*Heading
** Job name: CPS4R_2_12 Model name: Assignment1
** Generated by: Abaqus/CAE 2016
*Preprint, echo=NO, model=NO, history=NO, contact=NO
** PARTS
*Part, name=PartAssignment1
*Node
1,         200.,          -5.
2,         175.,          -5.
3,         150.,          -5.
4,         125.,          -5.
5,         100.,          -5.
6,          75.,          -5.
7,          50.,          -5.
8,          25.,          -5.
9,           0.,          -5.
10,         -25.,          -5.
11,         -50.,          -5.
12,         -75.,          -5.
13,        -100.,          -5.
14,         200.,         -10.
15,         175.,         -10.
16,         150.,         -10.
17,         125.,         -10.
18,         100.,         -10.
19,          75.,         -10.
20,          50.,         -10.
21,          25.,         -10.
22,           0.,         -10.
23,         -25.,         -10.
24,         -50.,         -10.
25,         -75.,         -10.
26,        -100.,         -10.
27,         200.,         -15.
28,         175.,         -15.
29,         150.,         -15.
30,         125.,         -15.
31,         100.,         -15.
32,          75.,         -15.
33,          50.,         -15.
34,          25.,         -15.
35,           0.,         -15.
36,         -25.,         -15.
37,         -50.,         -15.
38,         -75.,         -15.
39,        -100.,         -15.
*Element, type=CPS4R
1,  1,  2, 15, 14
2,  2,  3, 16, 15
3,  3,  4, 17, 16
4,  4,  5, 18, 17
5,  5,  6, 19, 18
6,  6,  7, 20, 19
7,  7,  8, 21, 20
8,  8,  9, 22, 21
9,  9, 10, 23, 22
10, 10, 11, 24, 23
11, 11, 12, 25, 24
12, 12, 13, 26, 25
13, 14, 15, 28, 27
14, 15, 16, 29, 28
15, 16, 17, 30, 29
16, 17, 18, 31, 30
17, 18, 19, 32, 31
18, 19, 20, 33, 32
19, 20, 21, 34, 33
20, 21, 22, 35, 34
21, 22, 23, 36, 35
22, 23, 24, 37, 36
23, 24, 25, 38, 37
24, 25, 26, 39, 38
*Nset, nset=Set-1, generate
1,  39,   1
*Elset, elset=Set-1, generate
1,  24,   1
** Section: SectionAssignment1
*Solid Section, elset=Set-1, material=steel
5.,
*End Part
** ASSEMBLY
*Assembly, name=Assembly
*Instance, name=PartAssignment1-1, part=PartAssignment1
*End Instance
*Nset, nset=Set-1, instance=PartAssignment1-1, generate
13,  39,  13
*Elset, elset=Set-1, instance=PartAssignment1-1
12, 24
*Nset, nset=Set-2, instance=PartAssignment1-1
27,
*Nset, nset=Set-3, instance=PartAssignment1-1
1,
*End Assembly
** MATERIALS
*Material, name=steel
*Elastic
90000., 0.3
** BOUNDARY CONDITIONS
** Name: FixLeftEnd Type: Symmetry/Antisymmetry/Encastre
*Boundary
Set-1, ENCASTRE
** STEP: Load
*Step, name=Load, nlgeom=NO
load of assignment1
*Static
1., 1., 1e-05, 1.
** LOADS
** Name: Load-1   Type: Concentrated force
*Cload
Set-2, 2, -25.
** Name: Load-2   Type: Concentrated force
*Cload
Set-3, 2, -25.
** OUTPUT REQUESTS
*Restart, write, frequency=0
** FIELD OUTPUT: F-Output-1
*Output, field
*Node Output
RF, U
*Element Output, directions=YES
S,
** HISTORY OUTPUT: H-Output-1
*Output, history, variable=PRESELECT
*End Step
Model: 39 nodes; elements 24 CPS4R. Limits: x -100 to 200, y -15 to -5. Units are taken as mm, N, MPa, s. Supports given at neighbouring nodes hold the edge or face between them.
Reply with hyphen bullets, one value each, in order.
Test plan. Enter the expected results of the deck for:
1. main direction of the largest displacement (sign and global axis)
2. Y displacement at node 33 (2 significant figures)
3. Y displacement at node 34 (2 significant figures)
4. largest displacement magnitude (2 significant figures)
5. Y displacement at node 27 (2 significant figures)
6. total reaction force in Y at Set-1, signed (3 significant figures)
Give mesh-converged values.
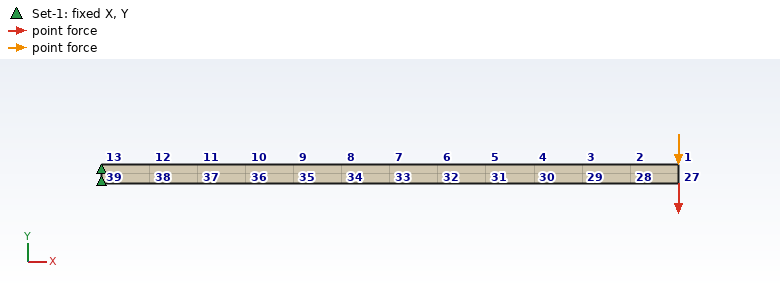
- -Y
- -3.7 mm
- -2.7 mm
- 12 mm
- -12 mm
- 50.0 N
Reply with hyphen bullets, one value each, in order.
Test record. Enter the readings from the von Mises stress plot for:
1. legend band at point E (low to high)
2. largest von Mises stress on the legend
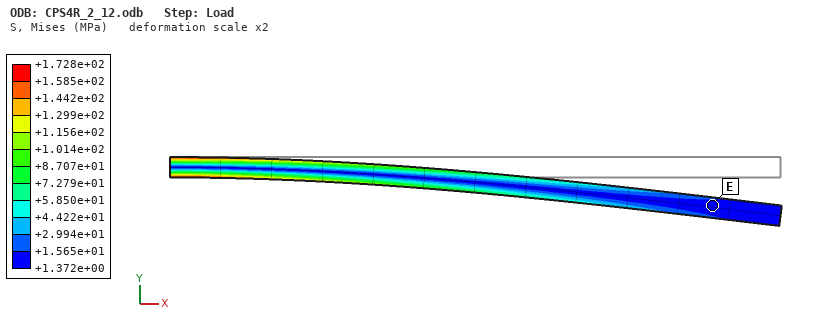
- +1.372e+00 to +1.565e+01 MPa
- +1.728e+02 MPa
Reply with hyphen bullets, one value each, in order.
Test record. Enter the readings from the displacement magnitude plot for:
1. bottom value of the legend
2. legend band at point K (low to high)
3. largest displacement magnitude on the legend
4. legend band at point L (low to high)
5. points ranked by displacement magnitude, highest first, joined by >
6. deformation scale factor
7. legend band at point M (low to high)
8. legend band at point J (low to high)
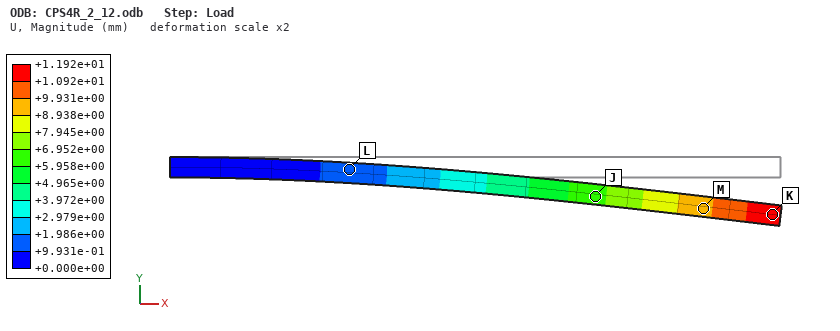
- +0.000e+00 mm
- +1.092e+01 to +1.192e+01 mm
- +1.192e+01 mm
- +9.931e-01 to +1.986e+00 mm
- K > M > J > L
- 2
- +8.938e+00 to +9.931e+00 mm
- +5.958e+00 to +6.952e+00 mm
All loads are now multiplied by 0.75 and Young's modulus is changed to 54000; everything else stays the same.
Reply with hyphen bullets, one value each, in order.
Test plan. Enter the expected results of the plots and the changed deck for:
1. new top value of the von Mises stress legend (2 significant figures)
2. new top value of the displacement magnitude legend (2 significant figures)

- 130 MPa
- 15 mm
